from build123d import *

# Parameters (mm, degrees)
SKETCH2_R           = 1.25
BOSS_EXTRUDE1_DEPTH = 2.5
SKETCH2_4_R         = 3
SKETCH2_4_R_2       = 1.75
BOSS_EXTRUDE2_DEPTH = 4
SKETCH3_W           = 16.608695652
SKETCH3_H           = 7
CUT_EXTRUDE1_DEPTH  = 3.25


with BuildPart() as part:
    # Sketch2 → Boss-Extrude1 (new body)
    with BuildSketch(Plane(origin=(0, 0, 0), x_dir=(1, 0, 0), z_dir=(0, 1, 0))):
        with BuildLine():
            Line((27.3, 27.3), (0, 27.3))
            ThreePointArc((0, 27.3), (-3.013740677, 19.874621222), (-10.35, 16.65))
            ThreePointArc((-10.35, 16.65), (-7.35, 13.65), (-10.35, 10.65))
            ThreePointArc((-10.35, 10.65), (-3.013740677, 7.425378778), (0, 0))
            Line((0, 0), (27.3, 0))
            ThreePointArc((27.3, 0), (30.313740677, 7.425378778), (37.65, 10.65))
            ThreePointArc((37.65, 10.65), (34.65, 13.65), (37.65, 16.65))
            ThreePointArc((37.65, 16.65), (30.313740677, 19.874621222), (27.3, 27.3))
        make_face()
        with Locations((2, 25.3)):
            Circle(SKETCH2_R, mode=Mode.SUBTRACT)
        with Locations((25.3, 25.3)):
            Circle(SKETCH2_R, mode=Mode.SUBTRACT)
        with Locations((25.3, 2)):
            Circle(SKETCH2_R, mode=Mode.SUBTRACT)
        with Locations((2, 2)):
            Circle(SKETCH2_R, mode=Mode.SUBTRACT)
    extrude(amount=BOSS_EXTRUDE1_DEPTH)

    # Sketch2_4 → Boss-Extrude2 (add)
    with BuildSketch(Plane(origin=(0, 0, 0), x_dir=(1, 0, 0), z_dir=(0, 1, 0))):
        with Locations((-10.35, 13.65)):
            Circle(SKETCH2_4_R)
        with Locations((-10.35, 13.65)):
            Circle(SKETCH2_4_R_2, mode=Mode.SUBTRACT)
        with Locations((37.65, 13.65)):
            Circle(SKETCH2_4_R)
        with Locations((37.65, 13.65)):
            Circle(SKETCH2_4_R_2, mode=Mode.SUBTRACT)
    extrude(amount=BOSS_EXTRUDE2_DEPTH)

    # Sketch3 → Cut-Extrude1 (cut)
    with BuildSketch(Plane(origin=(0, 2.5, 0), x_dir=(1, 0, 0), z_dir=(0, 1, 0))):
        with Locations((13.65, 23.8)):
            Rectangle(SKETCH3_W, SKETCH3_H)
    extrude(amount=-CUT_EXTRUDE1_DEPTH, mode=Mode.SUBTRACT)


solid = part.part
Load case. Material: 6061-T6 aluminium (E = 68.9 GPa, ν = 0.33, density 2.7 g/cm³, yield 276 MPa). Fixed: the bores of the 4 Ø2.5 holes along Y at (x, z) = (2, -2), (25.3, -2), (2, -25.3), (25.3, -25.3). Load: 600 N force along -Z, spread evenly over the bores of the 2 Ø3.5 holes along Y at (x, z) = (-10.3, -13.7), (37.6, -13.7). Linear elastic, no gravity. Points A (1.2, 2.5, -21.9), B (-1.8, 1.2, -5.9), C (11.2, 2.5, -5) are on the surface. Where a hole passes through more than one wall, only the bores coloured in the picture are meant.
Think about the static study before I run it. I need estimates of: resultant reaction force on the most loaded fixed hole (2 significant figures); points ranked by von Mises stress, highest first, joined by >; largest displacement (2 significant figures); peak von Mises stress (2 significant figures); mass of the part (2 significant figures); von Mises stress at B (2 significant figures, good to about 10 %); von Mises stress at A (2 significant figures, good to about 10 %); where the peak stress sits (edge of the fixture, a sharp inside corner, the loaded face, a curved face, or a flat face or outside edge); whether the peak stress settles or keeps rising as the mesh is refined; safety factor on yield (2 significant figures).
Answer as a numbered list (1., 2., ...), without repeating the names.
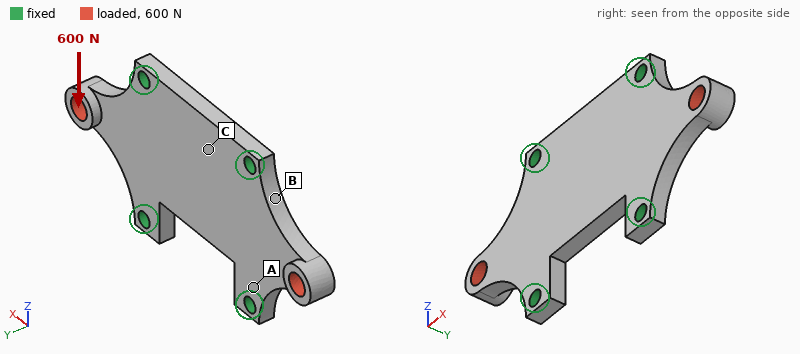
1. 210 N
2. B > A > C
3. 28 µm
4. 110 MPa
5. 5.8 g
6. 39 MPa
7. 17 MPa
8. a curved face
9. settles
10. 2.6
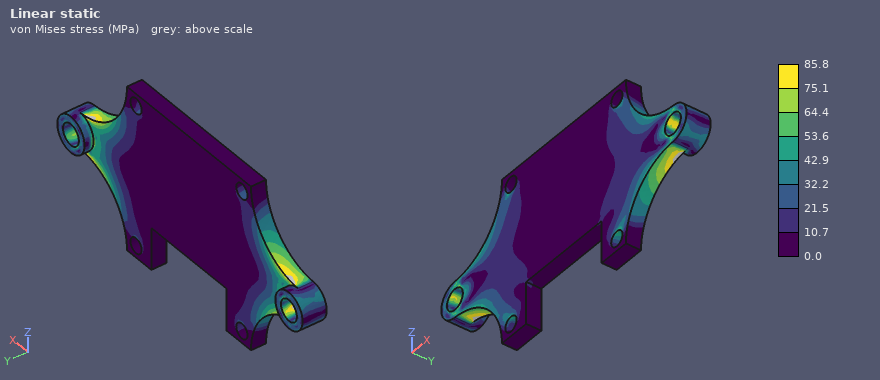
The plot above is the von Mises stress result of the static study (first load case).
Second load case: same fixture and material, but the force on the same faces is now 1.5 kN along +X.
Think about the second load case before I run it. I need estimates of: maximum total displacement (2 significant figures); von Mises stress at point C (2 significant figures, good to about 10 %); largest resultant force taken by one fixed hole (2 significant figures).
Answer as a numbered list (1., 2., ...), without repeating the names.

1. 89 µm
2. 14 MPa
3. 480 N
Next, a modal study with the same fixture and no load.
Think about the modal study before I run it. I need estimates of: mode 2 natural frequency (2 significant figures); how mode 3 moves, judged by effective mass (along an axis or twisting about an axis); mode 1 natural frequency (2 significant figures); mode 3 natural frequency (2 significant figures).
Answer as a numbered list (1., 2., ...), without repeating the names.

1. 9200 Hz
2. along Y
3. 8900 Hz
4. 15 kHz
